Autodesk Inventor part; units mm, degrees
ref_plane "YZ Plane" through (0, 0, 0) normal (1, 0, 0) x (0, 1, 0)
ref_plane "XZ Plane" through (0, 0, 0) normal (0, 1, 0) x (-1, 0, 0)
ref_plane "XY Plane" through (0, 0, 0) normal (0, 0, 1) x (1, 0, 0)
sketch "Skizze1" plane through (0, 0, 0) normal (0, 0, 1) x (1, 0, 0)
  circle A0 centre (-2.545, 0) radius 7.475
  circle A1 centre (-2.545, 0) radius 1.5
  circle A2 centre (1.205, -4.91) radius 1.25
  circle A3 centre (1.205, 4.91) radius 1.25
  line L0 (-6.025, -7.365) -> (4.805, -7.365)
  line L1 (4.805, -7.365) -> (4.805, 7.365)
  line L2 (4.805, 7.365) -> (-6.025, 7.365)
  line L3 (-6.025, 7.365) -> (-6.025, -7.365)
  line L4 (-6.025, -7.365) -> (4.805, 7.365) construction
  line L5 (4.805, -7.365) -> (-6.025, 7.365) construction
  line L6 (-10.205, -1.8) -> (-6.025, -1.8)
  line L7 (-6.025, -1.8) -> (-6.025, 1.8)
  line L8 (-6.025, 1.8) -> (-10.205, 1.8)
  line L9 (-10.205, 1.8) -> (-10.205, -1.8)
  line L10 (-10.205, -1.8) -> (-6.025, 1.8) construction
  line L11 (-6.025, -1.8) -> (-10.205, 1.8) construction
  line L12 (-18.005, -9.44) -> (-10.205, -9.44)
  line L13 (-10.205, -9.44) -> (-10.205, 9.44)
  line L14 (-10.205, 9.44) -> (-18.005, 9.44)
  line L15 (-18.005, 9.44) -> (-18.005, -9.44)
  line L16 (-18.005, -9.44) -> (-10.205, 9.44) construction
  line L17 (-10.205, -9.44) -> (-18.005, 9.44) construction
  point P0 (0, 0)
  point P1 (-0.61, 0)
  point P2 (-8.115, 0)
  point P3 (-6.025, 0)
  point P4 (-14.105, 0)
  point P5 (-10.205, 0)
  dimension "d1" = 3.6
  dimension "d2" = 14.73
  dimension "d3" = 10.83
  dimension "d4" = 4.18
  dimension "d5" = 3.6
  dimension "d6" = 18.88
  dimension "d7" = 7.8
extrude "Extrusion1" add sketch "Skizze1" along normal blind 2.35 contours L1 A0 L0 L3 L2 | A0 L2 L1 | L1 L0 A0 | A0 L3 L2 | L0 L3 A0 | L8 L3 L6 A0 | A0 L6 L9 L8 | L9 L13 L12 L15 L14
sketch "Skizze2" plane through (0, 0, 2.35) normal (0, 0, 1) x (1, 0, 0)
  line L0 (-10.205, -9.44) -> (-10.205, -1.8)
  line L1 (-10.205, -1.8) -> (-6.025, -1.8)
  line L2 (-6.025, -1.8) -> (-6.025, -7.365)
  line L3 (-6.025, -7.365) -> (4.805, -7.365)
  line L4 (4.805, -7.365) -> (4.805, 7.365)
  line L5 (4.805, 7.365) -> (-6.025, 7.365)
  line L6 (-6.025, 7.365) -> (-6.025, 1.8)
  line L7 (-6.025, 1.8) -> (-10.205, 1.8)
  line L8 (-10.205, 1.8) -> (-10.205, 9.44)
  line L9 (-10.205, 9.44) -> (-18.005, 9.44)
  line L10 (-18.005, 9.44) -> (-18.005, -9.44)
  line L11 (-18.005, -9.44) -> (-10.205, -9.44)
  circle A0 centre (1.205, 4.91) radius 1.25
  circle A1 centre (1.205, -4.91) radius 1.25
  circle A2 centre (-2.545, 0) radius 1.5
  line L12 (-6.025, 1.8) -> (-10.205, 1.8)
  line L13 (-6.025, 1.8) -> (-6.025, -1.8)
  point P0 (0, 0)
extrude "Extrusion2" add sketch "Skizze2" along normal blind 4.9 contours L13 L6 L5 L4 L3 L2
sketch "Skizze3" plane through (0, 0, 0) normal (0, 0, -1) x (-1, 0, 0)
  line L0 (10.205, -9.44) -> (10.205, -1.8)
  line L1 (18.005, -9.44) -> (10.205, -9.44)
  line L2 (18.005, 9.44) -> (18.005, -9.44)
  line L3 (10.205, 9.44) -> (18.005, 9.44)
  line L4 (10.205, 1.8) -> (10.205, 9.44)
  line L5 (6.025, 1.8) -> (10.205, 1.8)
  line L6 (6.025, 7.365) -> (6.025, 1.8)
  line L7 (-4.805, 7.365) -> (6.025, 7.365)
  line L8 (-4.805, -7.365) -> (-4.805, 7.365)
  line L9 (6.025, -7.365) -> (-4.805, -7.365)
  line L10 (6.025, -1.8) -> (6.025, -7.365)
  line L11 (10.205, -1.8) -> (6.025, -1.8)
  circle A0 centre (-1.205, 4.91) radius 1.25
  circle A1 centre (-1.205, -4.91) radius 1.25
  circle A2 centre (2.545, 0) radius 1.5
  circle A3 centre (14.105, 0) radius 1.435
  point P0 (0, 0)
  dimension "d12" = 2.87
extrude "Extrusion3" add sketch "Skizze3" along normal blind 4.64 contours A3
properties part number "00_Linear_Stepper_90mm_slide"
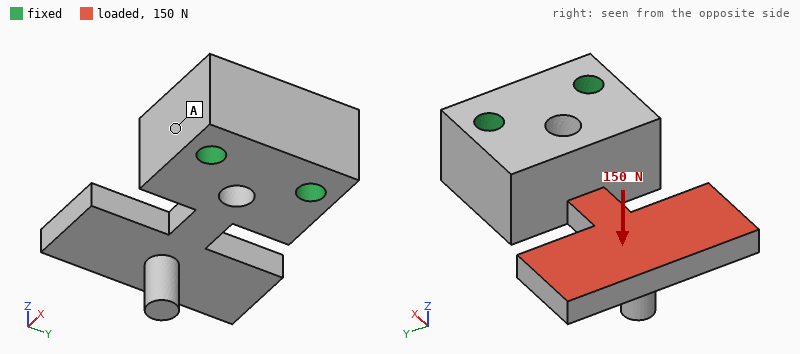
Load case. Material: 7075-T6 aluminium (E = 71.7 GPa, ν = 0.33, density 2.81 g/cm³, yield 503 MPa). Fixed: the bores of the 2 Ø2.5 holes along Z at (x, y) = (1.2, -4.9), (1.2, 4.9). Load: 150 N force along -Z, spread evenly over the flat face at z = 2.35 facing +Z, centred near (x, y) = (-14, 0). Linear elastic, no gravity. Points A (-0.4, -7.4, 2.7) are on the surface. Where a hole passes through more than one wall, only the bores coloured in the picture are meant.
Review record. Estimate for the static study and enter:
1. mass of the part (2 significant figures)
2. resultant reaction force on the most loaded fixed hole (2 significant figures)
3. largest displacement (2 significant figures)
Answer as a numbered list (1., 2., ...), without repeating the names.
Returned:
1. 4.1 g
2. 75 N
3. 0.22 mm
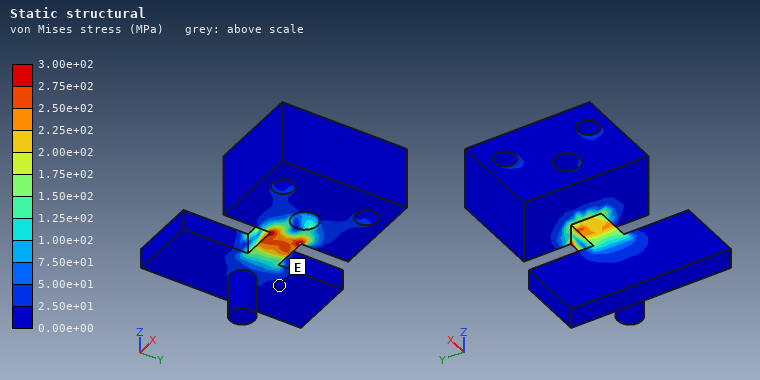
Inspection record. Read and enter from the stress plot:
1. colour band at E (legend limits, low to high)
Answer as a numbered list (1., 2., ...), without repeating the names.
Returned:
1. 0.00e+00 to 2.50e+01 MPa
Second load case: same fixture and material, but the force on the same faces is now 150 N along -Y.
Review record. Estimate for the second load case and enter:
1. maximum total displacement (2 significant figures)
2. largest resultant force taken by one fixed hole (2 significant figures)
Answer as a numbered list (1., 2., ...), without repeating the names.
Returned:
1. 0.14 mm
2. 230 N
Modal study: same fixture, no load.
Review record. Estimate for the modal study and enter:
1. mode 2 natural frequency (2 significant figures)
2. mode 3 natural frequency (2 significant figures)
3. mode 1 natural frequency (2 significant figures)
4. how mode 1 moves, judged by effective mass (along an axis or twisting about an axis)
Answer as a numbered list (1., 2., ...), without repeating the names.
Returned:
1. 5700 Hz
2. 5900 Hz
3. 4600 Hz
4. along Z
